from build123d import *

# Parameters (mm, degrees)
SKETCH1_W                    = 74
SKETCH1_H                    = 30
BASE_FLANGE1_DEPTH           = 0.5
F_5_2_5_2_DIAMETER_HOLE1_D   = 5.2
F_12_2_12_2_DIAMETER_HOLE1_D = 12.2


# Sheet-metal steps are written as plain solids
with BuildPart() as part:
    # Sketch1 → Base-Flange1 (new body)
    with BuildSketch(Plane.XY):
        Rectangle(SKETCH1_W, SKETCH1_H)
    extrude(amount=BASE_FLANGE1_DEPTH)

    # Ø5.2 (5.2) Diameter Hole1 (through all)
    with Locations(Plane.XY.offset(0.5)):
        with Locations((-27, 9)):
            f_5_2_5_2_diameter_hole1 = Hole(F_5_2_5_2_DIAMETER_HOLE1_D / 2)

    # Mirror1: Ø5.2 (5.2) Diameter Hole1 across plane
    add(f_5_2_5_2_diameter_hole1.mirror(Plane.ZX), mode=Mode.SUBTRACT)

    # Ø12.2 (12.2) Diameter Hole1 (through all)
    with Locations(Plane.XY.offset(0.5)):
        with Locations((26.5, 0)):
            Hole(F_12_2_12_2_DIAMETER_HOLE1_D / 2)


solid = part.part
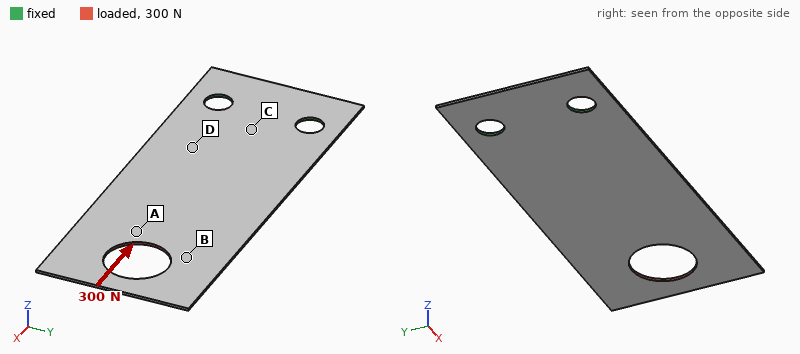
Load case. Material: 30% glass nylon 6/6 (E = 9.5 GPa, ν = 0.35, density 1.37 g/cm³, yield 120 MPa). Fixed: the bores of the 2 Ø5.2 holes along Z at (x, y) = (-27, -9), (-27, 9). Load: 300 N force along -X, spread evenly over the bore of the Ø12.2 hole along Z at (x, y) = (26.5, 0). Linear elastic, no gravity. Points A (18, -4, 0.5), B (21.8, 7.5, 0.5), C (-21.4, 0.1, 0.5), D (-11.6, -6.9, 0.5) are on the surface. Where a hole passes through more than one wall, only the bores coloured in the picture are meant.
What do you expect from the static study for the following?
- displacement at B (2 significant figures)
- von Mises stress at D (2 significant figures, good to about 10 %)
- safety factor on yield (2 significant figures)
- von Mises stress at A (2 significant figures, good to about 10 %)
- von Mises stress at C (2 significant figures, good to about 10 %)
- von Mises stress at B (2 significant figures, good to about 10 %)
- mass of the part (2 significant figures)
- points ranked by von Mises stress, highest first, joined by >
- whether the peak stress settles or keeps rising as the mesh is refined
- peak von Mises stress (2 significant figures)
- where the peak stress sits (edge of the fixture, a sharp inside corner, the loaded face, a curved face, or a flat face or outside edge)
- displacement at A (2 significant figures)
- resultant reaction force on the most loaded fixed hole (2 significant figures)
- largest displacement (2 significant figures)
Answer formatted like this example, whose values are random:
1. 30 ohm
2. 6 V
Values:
1. 0.11 mm
2. 20 MPa
3. 1.9
4. 26 MPa
5. 12 MPa
6. 34 MPa
7. 1.4 g
8. B > A > D > C
9. settles
10. 65 MPa
11. the loaded face
12. 0.094 mm
13. 150 N
14. 0.19 mm
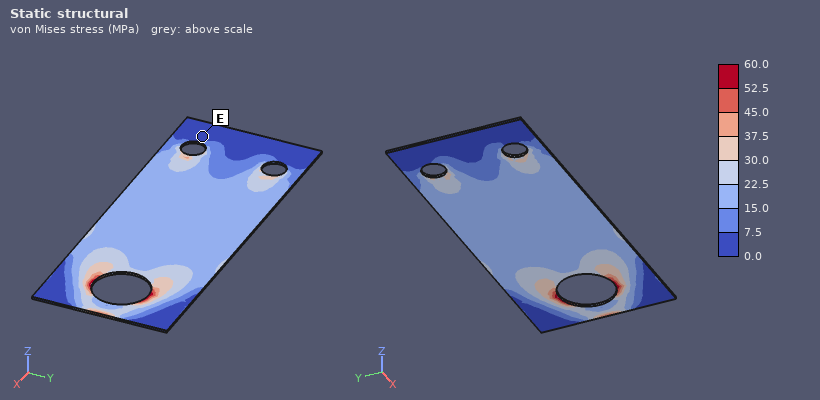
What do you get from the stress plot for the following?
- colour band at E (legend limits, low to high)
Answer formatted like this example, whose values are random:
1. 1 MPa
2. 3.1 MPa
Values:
1. 0.0 to 7.5 MPa
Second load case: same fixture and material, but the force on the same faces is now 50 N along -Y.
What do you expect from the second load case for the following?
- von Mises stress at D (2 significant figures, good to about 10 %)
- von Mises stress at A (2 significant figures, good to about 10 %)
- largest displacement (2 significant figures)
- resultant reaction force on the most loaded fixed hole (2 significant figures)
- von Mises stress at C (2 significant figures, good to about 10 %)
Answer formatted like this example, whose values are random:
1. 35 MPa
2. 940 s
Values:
1. 14 MPa
2. 9.3 MPa
3. 0.41 mm
4. 130 N
5. 7.1 MPa
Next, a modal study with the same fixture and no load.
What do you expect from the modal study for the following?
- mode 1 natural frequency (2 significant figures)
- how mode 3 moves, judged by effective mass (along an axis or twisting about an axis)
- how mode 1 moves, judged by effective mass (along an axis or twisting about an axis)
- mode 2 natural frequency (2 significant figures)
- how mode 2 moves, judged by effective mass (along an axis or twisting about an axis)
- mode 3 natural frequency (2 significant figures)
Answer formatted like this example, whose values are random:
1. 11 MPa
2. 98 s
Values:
1. 61 Hz
2. along Z
3. along Z
4. 240 Hz
5. twisting about X
6. 350 Hz
